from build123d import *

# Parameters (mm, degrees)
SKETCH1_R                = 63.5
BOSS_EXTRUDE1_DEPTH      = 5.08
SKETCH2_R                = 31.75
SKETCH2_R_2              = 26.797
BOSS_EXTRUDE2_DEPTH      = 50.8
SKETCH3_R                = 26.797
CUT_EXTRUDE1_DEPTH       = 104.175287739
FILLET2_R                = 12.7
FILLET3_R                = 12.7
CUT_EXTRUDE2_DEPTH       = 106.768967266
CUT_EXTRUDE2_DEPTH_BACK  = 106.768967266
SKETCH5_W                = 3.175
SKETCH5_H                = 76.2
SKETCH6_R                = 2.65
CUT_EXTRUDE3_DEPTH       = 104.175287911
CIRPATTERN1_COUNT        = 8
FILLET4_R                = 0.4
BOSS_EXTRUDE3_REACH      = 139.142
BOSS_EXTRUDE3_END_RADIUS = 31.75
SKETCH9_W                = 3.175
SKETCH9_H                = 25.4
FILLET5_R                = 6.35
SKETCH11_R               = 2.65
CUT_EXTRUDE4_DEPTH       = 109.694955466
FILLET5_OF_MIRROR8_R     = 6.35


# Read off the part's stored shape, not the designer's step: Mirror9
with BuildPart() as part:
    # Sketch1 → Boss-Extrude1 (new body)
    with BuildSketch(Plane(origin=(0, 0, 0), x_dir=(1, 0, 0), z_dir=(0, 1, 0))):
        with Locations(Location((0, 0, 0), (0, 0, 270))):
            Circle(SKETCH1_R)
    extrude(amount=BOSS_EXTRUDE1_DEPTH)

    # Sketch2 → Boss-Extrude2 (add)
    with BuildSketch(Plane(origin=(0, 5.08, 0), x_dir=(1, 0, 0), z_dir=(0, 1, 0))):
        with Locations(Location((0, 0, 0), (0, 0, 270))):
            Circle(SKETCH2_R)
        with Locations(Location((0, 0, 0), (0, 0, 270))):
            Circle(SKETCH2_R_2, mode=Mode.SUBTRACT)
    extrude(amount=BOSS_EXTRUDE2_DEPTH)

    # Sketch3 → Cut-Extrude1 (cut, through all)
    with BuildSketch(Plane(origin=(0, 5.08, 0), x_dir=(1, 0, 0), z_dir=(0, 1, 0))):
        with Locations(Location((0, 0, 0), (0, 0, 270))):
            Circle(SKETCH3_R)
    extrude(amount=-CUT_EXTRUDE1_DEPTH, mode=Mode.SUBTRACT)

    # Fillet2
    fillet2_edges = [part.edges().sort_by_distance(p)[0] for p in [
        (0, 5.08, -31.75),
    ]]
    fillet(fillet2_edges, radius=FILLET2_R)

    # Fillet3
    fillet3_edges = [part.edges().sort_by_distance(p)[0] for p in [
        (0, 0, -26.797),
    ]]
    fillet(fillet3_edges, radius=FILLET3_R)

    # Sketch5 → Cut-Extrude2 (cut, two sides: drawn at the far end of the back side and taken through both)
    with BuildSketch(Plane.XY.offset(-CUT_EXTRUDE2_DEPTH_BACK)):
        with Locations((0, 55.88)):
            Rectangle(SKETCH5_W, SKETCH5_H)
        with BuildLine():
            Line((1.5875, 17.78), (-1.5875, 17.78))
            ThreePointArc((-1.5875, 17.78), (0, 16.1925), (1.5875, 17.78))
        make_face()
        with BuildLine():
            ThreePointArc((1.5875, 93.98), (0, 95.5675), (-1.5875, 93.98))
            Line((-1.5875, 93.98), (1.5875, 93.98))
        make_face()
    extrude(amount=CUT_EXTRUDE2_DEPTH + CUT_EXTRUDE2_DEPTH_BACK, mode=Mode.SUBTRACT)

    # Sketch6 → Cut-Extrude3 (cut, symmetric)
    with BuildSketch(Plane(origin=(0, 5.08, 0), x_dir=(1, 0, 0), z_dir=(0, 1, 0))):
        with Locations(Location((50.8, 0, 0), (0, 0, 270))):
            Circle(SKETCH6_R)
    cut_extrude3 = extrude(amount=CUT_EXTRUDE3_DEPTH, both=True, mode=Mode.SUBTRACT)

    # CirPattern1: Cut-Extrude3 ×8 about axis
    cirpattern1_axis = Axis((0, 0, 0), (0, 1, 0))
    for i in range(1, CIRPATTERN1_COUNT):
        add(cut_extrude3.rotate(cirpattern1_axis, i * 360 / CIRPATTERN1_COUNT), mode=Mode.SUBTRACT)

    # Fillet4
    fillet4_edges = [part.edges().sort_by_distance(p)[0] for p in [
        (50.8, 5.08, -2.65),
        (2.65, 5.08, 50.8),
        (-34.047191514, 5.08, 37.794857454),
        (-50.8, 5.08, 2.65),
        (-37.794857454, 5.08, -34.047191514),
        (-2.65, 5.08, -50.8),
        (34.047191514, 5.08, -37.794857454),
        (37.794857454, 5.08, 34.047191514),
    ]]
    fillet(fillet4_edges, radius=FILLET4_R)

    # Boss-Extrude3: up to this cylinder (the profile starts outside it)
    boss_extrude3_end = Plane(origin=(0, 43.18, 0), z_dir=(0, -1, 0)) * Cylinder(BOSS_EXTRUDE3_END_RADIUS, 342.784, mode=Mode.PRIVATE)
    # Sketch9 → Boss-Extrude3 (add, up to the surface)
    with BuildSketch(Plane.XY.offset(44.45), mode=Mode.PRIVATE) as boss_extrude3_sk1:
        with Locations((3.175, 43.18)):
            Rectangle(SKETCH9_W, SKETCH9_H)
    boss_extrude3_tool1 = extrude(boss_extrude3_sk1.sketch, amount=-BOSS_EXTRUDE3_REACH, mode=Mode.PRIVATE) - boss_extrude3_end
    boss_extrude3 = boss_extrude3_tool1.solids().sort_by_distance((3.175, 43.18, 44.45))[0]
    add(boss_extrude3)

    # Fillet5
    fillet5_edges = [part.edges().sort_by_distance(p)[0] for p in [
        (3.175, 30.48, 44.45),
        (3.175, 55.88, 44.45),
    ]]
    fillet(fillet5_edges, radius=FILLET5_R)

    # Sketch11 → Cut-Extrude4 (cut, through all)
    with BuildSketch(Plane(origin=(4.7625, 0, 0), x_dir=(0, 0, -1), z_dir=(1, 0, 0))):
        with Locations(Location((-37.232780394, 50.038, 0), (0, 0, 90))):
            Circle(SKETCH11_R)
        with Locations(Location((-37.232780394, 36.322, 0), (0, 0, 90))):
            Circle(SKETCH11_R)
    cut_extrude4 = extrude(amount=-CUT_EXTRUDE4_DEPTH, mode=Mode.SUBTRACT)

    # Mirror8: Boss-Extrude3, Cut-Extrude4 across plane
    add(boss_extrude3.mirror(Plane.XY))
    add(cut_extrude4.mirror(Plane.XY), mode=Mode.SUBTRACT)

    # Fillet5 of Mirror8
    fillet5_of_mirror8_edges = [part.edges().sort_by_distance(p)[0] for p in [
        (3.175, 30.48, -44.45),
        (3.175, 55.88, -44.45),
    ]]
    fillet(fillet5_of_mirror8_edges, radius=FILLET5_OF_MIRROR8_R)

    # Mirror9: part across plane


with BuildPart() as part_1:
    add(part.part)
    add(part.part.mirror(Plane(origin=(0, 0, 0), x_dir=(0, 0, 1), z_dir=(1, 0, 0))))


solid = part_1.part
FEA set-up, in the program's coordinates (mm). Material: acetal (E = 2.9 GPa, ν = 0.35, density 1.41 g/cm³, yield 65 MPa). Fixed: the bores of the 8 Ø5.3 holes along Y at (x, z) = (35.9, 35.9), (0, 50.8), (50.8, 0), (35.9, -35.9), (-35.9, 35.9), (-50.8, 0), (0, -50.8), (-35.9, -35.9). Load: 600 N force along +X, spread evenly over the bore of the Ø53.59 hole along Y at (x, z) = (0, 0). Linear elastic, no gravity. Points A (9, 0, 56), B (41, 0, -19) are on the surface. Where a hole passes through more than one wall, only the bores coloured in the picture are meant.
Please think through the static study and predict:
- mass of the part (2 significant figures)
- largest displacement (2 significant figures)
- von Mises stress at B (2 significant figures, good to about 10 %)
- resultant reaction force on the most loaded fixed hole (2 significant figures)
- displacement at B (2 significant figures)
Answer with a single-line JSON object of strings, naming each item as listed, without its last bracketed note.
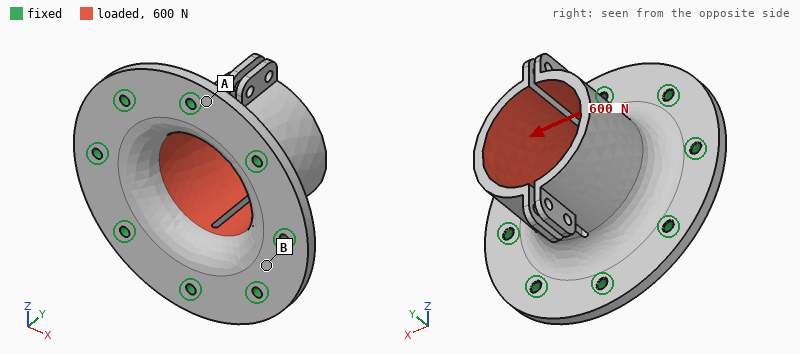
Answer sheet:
{"mass of the part": "140 g", "largest displacement": "0.16 mm", "von Mises stress at B": "1.3 MPa", "resultant reaction force on the most loaded fixed hole": "160 N", "displacement at B": "0.028 mm"}
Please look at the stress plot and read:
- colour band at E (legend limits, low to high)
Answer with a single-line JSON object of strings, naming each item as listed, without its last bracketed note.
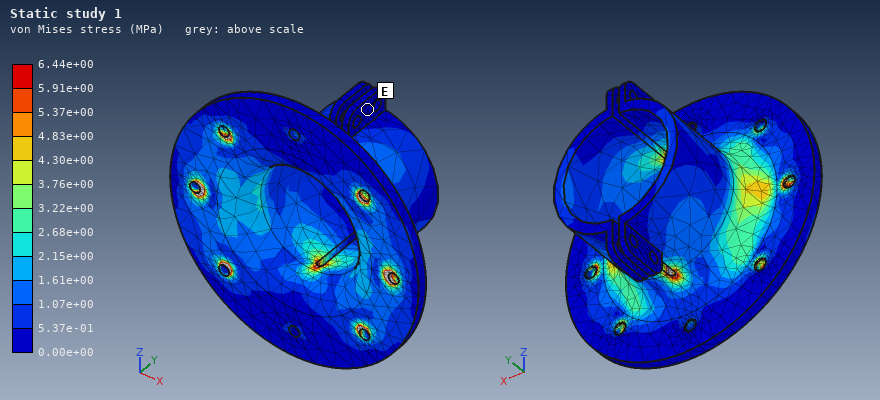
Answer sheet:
{"colour band at E": "0.00e+00 to 5.37e-01 MPa"}
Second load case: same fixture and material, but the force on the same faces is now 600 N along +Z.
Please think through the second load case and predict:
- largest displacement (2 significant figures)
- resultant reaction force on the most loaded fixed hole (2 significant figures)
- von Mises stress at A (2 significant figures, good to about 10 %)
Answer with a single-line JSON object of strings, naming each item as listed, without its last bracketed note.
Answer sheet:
{"largest displacement": "0.46 mm", "resultant reaction force on the most loaded fixed hole": "170 N", "von Mises stress at A": "1.0 MPa"}
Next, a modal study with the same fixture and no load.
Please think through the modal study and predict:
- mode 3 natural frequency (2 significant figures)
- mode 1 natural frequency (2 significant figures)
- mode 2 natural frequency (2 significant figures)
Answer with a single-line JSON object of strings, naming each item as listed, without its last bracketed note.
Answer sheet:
{"mode 3 natural frequency": "1000 Hz", "mode 1 natural frequency": "870 Hz", "mode 2 natural frequency": "870 Hz"}
